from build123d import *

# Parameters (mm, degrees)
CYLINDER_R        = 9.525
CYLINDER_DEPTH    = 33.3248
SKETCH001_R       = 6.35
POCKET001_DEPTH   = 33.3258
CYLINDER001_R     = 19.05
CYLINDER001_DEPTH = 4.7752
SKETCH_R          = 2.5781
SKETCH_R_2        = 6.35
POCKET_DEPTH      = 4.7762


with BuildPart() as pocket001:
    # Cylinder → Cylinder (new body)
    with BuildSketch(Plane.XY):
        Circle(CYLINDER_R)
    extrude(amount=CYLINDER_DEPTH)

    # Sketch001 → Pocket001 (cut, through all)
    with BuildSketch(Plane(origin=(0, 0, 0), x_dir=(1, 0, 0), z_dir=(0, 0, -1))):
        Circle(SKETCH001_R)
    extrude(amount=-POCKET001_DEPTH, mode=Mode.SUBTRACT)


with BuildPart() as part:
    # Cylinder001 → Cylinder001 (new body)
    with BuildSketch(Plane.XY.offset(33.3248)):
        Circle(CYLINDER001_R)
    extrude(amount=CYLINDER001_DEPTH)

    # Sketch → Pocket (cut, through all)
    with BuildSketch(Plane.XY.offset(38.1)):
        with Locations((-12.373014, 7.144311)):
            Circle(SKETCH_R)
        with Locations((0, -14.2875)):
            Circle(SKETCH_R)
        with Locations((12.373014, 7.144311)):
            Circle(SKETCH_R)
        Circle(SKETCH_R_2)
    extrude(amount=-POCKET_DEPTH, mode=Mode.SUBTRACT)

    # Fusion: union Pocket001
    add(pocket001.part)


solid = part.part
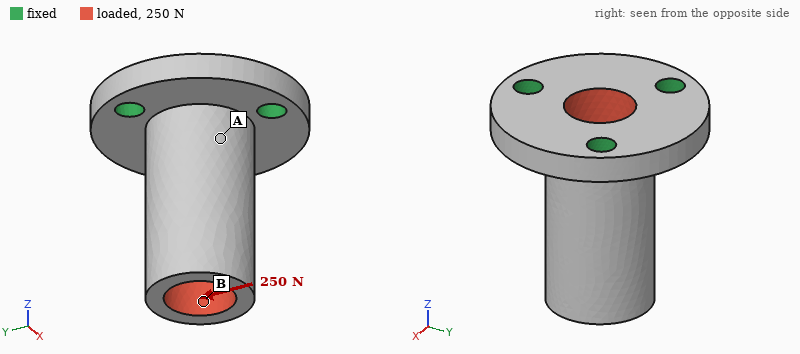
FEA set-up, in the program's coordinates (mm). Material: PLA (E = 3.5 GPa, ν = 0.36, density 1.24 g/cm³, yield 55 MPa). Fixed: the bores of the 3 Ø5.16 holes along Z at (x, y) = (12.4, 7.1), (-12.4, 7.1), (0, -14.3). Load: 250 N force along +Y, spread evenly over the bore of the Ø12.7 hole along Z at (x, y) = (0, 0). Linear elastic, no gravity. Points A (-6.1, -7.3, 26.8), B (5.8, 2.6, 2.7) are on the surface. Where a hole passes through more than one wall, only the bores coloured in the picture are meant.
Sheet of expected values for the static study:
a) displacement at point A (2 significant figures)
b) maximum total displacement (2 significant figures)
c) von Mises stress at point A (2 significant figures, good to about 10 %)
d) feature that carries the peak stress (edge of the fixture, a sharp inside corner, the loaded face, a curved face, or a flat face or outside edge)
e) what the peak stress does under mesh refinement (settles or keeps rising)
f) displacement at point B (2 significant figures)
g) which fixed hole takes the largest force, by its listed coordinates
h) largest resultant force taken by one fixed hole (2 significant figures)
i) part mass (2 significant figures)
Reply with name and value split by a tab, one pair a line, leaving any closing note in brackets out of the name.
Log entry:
displacement at point A	0.044 mm
maximum total displacement	0.18 mm
von Mises stress at point A	3.7 MPa
feature that carries the peak stress	edge of the fixture
what the peak stress does under mesh refinement	keeps rising
displacement at point B	0.16 mm
which fixed hole takes the largest force, by its listed coordinates	(0, -14.3)
largest resultant force taken by one fixed hole	230 N
part mass	12 g
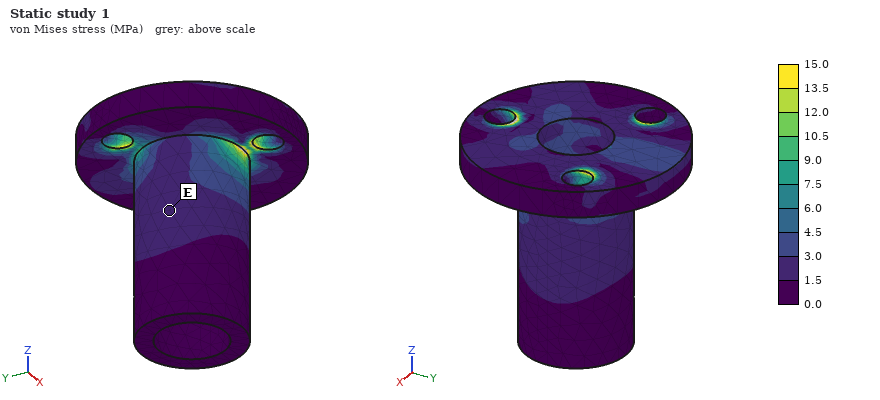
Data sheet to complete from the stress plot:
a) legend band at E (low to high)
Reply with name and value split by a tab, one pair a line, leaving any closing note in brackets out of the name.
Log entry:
legend band at E	1.5 to 3.0 MPa
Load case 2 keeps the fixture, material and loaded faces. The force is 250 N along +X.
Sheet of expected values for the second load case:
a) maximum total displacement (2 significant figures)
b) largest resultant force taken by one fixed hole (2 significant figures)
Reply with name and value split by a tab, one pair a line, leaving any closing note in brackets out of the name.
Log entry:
maximum total displacement	0.18 mm
largest resultant force taken by one fixed hole	200 N
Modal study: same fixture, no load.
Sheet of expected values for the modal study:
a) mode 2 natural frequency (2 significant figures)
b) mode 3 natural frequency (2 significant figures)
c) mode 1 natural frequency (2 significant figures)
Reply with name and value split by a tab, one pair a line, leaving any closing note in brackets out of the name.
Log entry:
mode 2 natural frequency	2600 Hz
mode 3 natural frequency	7100 Hz
mode 1 natural frequency	2600 Hz
